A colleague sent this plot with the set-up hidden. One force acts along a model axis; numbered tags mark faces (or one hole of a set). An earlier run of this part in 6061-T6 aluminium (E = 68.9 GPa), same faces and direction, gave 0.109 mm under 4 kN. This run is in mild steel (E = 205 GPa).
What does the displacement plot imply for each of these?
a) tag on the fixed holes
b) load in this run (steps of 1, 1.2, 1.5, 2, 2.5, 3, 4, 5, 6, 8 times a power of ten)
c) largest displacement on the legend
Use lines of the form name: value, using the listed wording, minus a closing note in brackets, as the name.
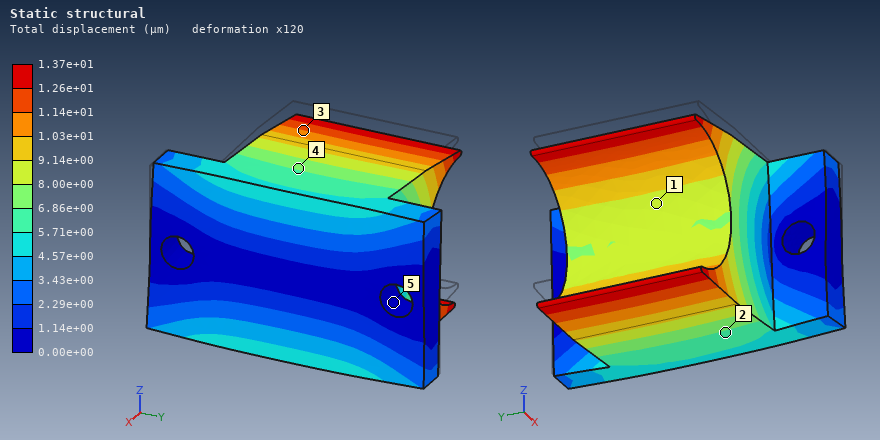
tag on the fixed holes: 5
load in this run: 1.5 kN
largest displacement on the legend: 1.37e+01 µm
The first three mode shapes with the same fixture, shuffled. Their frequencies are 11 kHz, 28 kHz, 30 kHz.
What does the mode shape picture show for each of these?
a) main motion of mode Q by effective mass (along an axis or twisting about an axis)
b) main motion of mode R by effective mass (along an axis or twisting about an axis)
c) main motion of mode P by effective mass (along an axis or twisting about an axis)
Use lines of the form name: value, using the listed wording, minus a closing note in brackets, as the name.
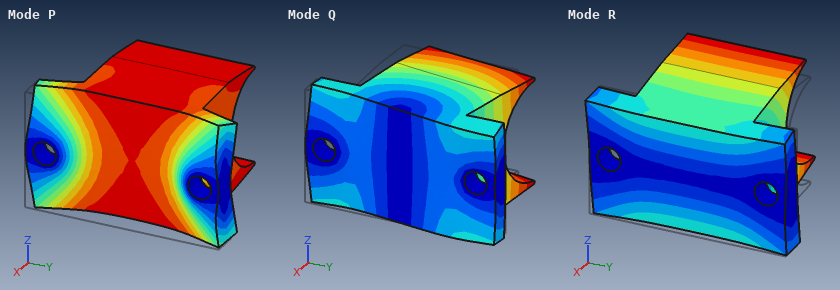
main motion of mode Q by effective mass: along Y
main motion of mode R by effective mass: along Z
main motion of mode P by effective mass: along X
